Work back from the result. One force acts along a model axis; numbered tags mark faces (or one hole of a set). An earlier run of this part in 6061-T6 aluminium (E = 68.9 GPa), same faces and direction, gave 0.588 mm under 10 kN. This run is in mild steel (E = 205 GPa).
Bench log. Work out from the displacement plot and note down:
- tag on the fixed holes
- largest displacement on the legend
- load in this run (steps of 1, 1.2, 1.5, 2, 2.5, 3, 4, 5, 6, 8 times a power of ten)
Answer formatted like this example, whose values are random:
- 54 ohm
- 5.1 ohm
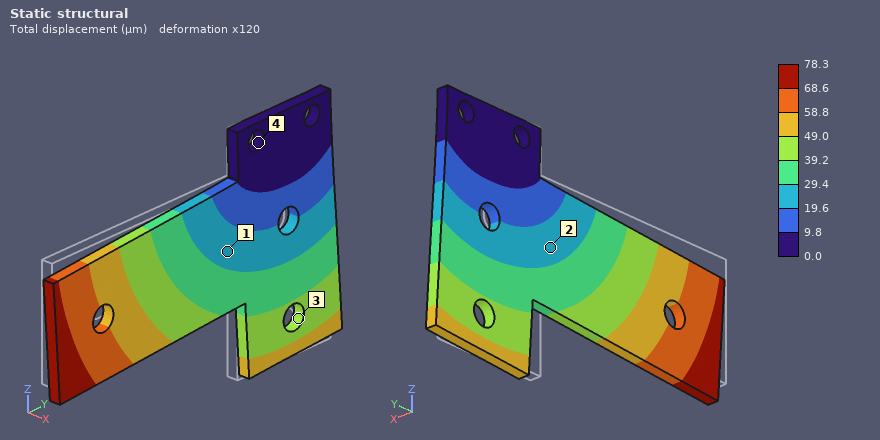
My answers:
- 4
- 78.3 µm
- 4 kN
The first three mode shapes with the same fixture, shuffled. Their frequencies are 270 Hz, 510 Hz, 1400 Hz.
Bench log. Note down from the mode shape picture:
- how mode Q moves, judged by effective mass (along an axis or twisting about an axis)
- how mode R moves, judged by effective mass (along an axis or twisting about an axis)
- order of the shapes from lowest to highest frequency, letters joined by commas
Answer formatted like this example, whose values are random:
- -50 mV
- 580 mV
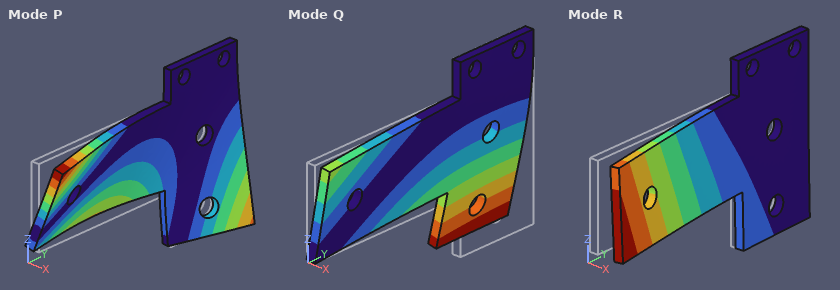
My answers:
- along X
- along X
- R, Q, P
